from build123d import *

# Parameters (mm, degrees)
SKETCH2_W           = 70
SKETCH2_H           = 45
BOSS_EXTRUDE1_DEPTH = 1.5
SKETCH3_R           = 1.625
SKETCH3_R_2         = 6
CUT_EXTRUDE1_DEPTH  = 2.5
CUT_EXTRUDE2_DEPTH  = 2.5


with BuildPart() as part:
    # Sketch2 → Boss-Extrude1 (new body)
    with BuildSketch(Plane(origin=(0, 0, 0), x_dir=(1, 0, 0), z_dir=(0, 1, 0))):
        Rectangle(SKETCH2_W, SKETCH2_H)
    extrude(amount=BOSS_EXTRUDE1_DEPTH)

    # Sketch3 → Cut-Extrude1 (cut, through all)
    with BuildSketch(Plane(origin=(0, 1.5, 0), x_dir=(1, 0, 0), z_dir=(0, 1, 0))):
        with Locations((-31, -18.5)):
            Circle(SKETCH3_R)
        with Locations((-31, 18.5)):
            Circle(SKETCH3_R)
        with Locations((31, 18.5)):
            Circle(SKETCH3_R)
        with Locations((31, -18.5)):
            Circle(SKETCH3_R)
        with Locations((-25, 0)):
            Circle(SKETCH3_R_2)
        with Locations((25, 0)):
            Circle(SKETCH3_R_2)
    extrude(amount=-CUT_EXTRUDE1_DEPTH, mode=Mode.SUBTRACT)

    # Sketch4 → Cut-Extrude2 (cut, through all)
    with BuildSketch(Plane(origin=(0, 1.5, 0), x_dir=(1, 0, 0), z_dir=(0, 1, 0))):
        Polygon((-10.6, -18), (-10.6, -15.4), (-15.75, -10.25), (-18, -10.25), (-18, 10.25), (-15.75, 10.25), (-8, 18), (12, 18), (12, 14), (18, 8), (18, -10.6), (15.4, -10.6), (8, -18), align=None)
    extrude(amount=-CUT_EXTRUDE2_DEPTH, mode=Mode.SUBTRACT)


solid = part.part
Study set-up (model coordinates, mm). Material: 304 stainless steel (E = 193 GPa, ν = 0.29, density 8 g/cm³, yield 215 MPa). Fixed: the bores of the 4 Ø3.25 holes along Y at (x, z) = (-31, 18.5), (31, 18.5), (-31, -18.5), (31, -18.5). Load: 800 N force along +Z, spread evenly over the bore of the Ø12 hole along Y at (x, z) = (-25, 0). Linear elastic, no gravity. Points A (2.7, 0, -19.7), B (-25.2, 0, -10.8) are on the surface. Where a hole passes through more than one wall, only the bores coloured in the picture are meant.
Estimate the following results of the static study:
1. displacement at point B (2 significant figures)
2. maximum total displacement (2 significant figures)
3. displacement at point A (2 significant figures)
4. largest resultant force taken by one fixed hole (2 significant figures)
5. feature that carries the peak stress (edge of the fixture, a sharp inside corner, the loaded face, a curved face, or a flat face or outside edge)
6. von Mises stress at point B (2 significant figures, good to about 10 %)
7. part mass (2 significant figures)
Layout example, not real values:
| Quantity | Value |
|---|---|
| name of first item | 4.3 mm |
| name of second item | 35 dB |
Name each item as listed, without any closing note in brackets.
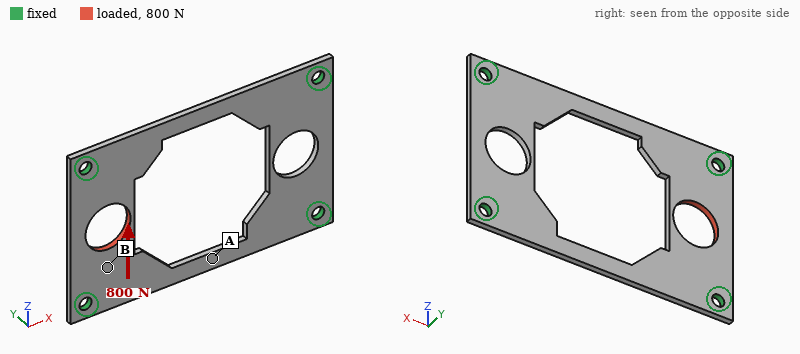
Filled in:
| Quantity | Value |
|---|---|
| displacement at point B | 2.3 µm |
| maximum total displacement | 5.2 µm |
| displacement at point A | 2.8 µm |
| largest resultant force taken by one fixed hole | 400 N |
| feature that carries the peak stress | edge of the fixture |
| von Mises stress at point B | 20 MPa |
| part mass | 21 g |
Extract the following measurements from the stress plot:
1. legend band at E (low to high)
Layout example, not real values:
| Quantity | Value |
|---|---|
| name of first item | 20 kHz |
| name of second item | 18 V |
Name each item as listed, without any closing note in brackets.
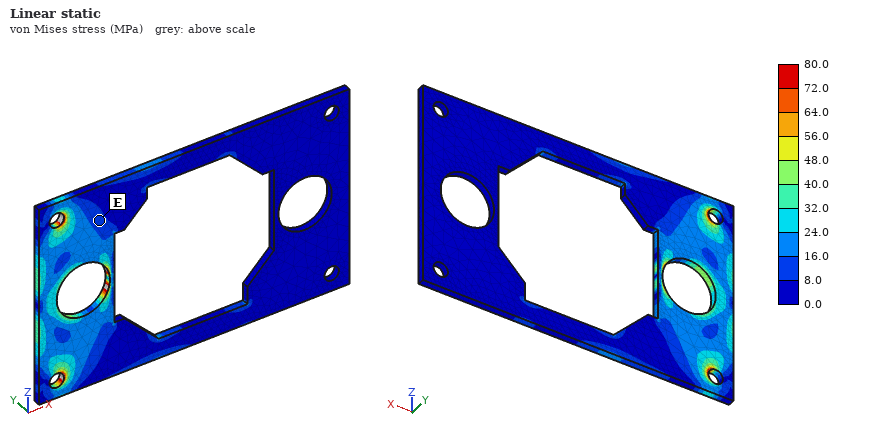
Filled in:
| Quantity | Value |
|---|---|
| legend band at E | 8.0 to 16.0 MPa |
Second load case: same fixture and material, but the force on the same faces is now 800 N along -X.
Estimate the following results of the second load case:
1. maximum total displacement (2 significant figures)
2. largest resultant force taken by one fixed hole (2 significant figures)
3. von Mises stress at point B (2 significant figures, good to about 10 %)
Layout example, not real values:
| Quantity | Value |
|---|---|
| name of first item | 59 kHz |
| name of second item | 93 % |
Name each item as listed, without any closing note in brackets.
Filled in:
| Quantity | Value |
|---|---|
| maximum total displacement | 10 µm |
| largest resultant force taken by one fixed hole | 420 N |
| von Mises stress at point B | 38 MPa |
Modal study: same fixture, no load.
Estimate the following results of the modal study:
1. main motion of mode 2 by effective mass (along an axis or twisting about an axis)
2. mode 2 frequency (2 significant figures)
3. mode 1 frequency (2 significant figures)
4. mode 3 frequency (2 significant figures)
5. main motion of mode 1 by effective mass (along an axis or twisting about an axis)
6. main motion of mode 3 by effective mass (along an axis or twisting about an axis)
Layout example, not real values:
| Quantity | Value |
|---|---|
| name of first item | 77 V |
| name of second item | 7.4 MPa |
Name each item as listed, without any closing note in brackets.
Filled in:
| Quantity | Value |
|---|---|
| main motion of mode 2 by effective mass | twisting about X |
| mode 2 frequency | 2700 Hz |
| mode 1 frequency | 2500 Hz |
| mode 3 frequency | 4700 Hz |
| main motion of mode 1 by effective mass | along Y |
| main motion of mode 3 by effective mass | twisting about Z |
